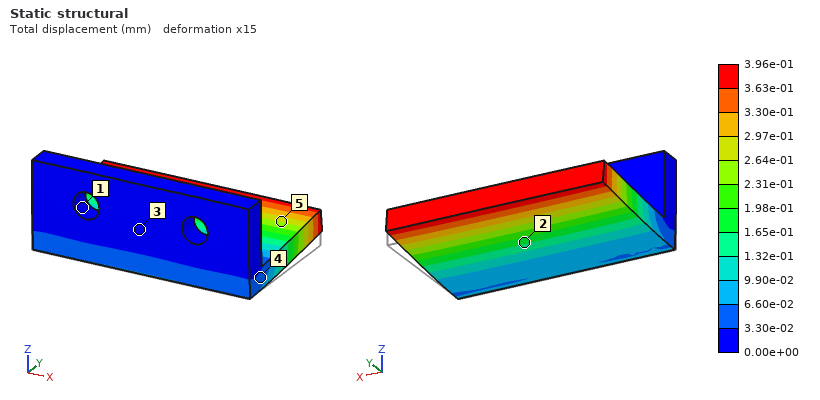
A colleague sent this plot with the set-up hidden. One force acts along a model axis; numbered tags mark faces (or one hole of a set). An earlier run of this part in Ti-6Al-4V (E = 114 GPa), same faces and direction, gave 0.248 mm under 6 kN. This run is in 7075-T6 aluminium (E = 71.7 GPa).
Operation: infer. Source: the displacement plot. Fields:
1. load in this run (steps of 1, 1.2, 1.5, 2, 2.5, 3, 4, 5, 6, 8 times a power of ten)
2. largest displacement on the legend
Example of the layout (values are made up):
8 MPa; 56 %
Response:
6 kN; 3.96e-01 mm
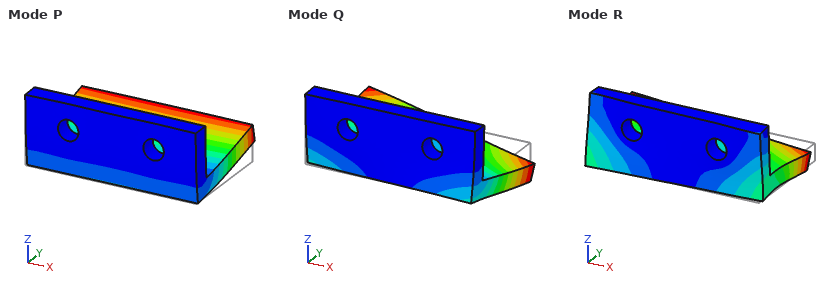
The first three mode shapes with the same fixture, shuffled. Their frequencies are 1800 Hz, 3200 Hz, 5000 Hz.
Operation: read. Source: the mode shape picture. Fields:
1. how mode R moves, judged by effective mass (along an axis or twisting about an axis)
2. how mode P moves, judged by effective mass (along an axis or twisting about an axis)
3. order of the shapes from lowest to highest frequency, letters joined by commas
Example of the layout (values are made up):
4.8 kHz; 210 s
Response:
along X; along Z; P, Q, R
